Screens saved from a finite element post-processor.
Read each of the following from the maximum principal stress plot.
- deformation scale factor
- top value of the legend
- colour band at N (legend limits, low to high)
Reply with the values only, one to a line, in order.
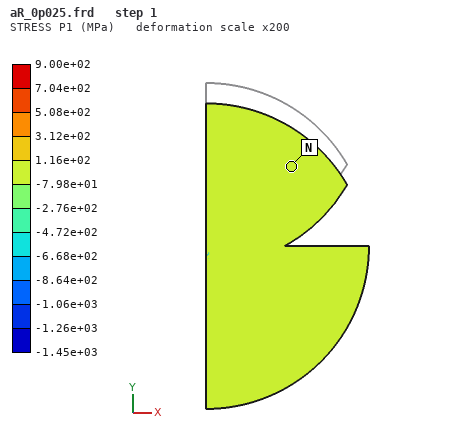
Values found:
200
9.00e+02 MPa
-7.98e+01 to 1.16e+02 MPa
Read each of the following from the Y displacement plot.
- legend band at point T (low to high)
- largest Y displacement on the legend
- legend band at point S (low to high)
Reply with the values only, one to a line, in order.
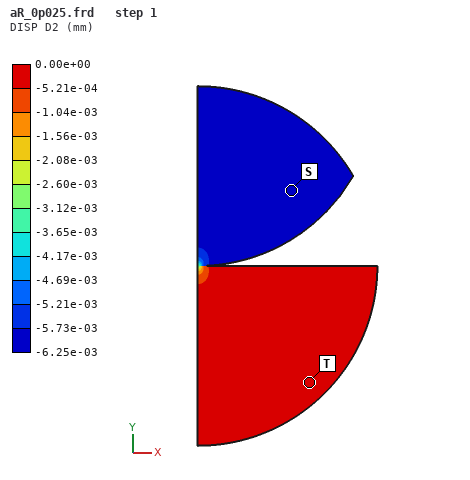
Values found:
-5.21e-04 to 0.00e+00 mm
0.00e+00 mm
-6.25e-03 to -5.73e-03 mm
